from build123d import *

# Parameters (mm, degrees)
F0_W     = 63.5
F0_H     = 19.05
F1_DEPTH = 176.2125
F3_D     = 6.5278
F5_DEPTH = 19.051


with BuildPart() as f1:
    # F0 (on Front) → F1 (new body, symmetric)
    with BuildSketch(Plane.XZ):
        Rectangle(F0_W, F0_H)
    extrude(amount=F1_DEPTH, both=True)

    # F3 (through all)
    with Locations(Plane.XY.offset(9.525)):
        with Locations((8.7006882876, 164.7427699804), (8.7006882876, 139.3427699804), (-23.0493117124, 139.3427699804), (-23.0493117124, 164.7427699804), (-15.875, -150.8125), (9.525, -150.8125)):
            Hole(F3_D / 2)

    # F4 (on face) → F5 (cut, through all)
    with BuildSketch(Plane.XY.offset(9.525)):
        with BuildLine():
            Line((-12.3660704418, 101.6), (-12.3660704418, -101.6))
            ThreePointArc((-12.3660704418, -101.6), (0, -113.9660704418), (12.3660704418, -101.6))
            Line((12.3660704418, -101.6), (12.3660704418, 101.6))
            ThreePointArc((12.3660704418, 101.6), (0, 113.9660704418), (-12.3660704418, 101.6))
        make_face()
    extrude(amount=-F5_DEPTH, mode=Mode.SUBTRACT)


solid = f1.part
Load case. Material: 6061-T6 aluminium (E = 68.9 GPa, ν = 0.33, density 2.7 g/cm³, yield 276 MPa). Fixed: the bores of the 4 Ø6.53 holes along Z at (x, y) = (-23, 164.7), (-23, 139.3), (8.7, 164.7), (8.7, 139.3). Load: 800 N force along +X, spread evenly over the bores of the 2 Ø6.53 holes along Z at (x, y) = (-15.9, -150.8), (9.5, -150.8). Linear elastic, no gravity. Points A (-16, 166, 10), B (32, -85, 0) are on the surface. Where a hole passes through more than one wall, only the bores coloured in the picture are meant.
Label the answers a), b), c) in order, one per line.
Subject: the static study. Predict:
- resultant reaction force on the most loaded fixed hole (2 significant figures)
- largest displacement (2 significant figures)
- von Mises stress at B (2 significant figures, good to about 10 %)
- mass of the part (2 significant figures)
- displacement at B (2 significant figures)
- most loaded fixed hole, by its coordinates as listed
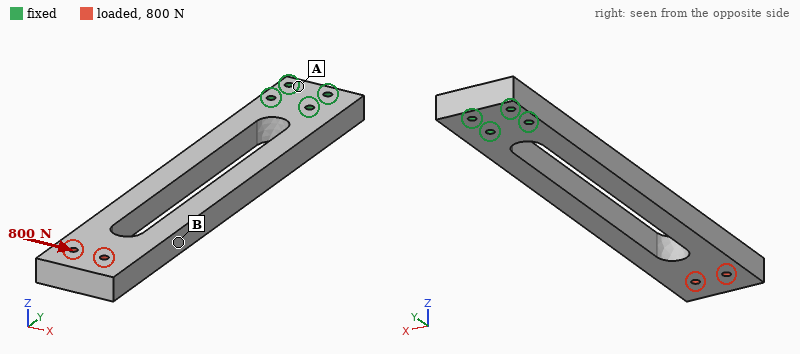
a) 5.0 kN
b) 0.82 mm
c) 18 MPa
d) 860 g
e) 0.67 mm
f) (-23, 139.3)
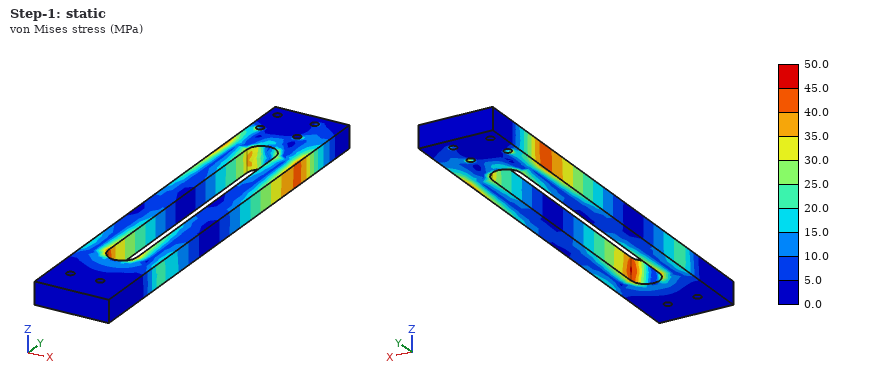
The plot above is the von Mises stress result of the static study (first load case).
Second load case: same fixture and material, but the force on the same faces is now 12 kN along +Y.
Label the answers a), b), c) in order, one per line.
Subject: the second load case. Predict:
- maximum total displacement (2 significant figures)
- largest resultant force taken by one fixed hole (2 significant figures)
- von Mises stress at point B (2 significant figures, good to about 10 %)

a) 92 µm
b) 5.0 kN
c) 11 MPa
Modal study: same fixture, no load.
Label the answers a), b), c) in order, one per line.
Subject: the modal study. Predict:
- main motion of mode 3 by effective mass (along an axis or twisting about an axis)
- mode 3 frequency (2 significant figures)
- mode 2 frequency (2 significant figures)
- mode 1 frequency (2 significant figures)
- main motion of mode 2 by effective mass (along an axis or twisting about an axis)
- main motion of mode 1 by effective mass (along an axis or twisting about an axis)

a) twisting about Y
b) 810 Hz
c) 280 Hz
d) 140 Hz
e) along X
f) along Z
